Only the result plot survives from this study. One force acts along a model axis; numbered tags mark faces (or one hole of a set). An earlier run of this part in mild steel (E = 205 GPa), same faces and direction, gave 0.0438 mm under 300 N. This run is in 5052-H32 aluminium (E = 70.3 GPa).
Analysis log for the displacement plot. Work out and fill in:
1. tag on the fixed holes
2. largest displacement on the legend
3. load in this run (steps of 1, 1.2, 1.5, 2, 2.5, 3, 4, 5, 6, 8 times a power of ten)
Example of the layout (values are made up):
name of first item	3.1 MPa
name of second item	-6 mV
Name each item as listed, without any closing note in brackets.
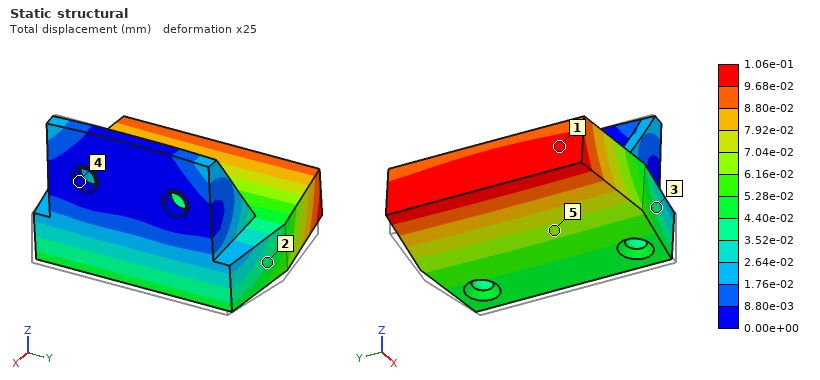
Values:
tag on the fixed holes	4
largest displacement on the legend	1.06e-01 mm
load in this run	250 N
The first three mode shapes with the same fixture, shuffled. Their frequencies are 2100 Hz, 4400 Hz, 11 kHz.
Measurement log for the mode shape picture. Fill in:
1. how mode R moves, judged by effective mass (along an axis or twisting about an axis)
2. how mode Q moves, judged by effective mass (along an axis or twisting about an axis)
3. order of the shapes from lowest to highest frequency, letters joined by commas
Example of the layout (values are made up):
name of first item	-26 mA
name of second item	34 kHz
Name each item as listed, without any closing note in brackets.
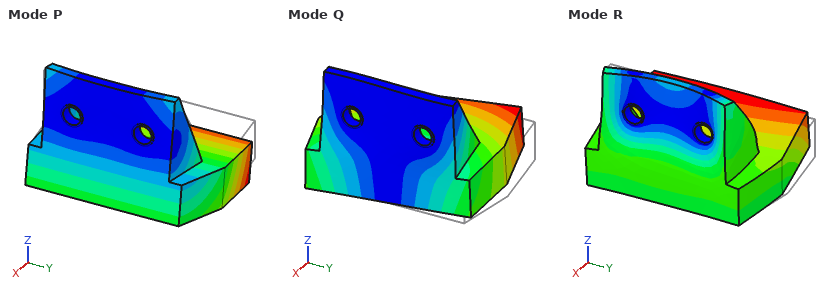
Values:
how mode R moves, judged by effective mass	along X
how mode Q moves, judged by effective mass	along Y
order of the shapes from lowest to highest frequency, letters joined by commas	P, Q, R
